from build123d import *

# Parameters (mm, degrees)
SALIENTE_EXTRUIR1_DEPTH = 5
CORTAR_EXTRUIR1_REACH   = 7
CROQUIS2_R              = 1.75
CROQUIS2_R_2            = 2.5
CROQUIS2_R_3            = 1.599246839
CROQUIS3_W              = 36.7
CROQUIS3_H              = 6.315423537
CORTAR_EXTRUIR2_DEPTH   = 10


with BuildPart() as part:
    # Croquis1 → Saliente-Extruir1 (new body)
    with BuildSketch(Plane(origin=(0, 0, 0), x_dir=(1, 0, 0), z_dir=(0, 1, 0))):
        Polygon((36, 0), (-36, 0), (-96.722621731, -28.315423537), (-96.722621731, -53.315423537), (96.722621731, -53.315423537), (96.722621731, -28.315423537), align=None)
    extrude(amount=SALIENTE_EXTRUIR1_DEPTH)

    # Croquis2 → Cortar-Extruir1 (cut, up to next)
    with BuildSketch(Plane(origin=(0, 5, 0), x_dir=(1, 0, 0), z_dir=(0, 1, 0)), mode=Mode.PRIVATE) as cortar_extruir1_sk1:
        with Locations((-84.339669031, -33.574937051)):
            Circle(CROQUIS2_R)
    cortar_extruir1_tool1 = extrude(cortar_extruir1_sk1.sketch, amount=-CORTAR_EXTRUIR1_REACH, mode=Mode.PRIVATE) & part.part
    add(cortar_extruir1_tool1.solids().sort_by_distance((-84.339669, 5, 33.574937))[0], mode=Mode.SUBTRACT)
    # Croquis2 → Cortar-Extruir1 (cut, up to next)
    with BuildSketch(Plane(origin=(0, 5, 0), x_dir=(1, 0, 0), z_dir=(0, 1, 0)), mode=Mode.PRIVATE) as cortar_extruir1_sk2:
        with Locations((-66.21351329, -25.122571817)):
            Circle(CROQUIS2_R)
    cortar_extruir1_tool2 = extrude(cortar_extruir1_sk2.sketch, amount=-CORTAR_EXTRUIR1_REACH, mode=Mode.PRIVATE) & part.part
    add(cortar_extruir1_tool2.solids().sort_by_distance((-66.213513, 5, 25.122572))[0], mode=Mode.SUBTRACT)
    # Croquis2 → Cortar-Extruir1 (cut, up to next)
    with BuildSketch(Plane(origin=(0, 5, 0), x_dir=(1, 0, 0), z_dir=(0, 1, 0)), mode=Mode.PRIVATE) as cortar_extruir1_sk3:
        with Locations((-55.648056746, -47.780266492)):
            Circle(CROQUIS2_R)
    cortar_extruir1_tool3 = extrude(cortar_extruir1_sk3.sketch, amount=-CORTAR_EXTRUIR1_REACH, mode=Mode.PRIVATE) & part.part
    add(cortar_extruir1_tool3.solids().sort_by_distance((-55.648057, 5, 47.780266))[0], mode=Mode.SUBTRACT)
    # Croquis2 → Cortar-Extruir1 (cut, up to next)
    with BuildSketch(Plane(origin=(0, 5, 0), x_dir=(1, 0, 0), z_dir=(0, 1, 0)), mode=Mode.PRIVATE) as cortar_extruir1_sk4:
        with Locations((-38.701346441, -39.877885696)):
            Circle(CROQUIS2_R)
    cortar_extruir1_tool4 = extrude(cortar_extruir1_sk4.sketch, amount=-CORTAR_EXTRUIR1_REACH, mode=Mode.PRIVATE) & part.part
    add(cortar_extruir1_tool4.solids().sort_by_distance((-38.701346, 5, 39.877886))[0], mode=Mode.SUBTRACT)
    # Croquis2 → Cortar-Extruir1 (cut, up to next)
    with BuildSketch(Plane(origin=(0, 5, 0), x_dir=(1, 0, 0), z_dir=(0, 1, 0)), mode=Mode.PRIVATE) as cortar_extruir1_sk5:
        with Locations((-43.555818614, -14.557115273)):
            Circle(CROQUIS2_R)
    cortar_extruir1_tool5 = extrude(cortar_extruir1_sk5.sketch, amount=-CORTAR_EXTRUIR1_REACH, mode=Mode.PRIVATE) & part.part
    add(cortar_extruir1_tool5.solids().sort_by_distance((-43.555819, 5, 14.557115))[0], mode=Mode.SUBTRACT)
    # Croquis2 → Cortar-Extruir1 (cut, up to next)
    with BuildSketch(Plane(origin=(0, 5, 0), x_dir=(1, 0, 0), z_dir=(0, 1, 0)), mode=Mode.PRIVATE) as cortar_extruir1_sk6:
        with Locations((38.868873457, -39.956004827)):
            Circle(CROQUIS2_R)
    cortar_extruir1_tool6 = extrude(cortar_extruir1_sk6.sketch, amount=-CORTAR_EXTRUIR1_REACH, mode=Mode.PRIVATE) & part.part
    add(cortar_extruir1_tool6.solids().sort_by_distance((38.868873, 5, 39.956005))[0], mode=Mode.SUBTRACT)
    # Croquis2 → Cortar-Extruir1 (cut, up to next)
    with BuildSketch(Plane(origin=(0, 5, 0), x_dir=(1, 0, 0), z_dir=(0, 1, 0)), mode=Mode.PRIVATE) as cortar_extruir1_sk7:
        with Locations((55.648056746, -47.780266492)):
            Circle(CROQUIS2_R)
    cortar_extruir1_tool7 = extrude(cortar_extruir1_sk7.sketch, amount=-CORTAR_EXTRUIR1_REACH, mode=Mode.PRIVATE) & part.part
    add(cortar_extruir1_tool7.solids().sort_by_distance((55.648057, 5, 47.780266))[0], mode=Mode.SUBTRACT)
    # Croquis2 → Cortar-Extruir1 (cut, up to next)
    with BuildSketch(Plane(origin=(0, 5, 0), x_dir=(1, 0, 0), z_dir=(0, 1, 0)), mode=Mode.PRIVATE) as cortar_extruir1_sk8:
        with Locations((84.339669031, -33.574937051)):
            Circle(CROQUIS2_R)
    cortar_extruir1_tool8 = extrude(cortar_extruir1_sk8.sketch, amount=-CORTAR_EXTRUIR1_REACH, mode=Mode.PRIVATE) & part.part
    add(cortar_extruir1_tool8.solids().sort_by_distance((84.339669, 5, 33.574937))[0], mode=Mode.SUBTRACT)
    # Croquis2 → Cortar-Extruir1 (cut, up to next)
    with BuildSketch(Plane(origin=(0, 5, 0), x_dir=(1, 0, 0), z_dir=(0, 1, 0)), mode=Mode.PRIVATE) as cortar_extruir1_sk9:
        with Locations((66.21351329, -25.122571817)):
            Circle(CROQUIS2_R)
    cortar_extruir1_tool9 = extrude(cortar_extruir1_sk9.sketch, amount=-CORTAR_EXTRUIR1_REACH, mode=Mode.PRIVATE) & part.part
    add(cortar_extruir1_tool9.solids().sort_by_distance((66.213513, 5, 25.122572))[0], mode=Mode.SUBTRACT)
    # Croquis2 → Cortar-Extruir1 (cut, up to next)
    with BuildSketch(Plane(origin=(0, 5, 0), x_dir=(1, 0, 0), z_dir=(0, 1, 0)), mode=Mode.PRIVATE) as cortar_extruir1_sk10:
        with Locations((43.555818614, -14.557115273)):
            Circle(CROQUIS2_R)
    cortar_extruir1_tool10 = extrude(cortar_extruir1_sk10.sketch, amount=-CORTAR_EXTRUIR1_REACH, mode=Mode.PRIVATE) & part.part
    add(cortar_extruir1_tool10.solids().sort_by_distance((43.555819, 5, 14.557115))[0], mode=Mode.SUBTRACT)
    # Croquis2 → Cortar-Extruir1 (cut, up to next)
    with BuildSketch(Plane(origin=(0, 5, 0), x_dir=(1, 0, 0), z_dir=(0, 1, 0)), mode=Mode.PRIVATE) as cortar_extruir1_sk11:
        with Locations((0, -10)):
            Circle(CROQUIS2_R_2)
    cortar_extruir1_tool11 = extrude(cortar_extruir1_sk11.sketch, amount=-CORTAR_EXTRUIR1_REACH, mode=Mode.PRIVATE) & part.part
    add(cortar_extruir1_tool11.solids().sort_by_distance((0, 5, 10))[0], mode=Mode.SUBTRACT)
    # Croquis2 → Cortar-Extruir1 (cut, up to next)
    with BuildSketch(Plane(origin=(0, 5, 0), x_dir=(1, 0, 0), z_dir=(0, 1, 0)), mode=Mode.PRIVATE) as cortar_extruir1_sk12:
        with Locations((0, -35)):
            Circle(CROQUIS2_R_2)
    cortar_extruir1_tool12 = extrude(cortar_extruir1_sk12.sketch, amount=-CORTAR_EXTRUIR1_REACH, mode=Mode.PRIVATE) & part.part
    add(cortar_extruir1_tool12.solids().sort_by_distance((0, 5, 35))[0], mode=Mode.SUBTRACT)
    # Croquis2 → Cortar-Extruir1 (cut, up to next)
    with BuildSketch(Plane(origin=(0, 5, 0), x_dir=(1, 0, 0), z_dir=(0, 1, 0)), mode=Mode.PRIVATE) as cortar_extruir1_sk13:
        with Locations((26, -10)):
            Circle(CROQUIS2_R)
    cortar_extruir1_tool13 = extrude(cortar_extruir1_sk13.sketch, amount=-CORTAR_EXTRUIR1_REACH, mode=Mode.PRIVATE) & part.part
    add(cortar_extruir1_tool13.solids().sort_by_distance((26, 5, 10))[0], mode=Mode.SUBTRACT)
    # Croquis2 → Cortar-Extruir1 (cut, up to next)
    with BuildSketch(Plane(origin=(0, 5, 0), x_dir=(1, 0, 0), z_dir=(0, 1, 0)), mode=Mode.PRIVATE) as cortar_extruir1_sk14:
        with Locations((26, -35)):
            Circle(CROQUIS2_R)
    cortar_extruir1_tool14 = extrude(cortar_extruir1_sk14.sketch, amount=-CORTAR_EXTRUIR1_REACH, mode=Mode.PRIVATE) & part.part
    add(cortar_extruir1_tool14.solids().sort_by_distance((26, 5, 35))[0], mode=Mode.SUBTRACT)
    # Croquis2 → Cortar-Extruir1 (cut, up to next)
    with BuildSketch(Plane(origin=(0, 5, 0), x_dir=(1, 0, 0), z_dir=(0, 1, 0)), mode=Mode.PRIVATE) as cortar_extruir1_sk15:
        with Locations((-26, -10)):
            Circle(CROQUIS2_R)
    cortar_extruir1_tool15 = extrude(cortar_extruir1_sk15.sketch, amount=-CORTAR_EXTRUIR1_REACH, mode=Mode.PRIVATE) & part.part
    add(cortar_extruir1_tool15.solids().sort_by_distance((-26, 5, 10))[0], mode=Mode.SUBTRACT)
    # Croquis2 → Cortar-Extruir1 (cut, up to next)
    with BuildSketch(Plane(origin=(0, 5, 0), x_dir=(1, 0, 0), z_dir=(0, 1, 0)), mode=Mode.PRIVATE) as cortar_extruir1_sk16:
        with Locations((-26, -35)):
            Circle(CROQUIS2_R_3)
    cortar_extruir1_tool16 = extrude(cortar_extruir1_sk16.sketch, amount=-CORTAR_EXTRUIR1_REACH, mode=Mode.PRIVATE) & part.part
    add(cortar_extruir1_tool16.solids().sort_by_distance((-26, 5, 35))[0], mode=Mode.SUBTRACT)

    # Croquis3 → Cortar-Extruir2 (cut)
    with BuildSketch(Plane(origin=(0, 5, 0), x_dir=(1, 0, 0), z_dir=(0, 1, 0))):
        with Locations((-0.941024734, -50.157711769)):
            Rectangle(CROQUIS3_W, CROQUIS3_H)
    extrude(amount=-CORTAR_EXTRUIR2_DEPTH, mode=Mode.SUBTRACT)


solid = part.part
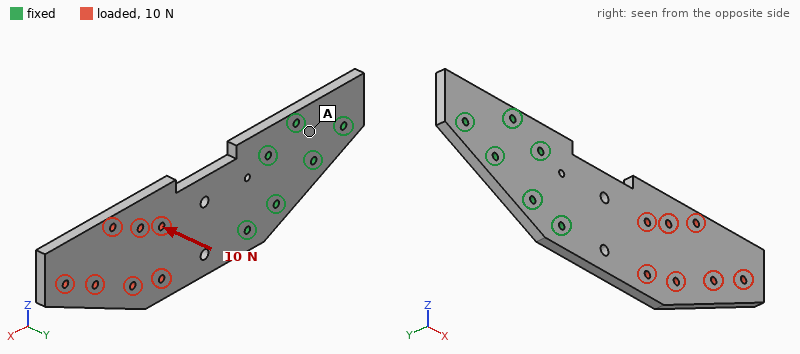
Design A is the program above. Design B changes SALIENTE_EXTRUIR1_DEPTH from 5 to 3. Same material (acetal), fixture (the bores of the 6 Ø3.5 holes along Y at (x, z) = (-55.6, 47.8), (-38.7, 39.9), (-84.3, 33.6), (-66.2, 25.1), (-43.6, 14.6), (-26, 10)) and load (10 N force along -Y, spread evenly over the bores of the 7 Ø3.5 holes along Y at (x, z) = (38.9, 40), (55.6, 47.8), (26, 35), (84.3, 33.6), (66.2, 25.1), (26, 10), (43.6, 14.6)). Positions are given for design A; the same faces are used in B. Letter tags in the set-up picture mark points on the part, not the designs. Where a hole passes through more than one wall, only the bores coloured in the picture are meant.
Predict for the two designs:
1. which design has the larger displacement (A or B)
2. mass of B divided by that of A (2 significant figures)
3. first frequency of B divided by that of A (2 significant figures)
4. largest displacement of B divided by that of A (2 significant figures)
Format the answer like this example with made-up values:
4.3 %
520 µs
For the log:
B
0.60
0.61
4.5
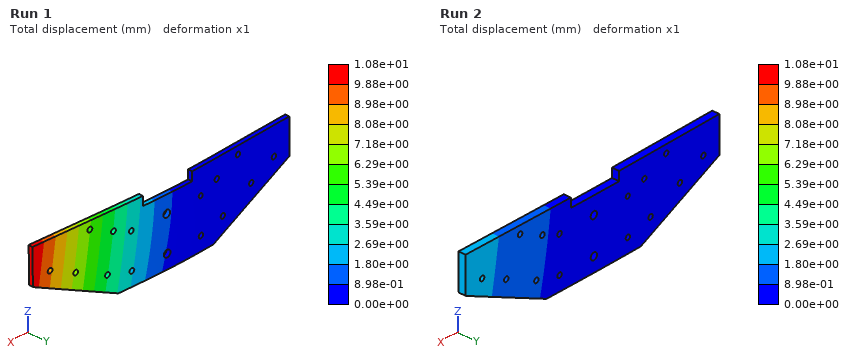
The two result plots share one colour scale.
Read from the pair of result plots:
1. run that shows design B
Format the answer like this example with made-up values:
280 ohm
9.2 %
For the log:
Run 1
